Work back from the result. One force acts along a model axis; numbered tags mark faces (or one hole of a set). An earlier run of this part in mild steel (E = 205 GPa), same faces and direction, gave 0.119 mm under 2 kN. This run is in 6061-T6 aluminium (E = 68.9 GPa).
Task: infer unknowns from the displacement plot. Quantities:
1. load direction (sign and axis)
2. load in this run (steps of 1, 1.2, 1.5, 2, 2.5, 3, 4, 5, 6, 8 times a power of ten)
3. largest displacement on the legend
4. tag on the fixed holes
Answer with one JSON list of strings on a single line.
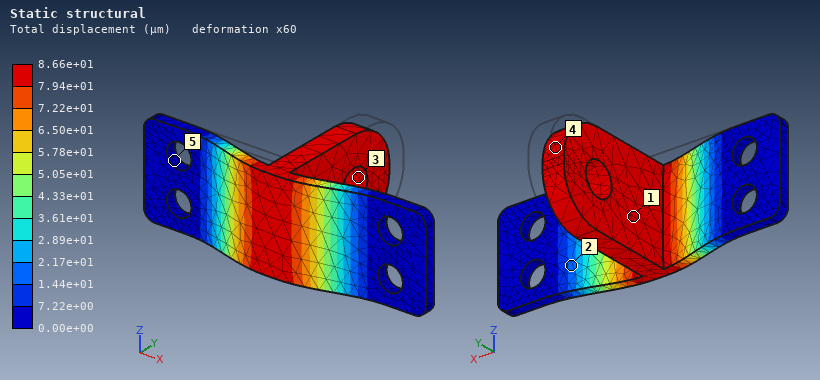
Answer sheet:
["-Y", "500 N", "8.66e+01 µm", "5"]
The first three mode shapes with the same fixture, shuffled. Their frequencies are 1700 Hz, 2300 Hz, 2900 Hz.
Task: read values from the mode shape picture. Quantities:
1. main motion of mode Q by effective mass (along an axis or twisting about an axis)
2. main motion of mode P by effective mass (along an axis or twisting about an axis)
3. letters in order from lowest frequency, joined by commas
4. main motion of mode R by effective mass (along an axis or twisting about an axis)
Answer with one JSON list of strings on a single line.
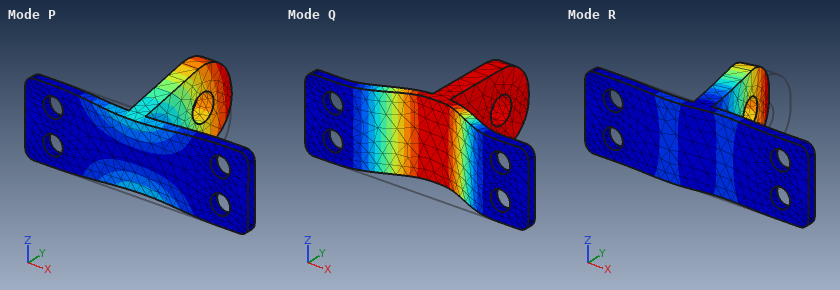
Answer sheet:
["along Y", "along Z", "P, R, Q", "along X"]
